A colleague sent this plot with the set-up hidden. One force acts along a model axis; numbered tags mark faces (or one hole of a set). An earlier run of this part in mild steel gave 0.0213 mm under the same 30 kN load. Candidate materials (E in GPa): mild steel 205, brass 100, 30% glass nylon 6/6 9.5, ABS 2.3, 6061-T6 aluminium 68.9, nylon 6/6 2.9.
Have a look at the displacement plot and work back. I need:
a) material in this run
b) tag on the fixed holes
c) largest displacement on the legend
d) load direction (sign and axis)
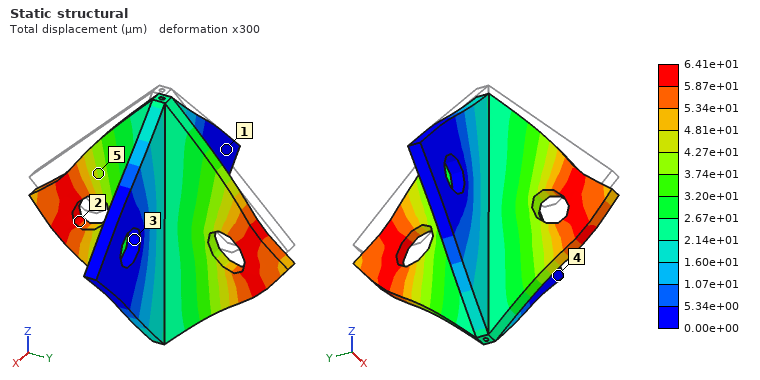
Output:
6061-T6 aluminium
3
6.41e+01 µm
-Z
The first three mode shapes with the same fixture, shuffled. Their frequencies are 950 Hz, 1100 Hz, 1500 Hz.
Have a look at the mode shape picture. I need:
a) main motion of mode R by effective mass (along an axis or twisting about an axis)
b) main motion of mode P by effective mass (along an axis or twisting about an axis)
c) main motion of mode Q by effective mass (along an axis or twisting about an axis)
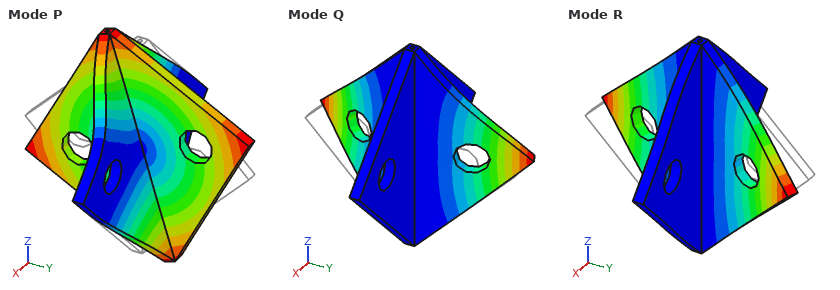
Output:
twisting about Z
twisting about X
along X
